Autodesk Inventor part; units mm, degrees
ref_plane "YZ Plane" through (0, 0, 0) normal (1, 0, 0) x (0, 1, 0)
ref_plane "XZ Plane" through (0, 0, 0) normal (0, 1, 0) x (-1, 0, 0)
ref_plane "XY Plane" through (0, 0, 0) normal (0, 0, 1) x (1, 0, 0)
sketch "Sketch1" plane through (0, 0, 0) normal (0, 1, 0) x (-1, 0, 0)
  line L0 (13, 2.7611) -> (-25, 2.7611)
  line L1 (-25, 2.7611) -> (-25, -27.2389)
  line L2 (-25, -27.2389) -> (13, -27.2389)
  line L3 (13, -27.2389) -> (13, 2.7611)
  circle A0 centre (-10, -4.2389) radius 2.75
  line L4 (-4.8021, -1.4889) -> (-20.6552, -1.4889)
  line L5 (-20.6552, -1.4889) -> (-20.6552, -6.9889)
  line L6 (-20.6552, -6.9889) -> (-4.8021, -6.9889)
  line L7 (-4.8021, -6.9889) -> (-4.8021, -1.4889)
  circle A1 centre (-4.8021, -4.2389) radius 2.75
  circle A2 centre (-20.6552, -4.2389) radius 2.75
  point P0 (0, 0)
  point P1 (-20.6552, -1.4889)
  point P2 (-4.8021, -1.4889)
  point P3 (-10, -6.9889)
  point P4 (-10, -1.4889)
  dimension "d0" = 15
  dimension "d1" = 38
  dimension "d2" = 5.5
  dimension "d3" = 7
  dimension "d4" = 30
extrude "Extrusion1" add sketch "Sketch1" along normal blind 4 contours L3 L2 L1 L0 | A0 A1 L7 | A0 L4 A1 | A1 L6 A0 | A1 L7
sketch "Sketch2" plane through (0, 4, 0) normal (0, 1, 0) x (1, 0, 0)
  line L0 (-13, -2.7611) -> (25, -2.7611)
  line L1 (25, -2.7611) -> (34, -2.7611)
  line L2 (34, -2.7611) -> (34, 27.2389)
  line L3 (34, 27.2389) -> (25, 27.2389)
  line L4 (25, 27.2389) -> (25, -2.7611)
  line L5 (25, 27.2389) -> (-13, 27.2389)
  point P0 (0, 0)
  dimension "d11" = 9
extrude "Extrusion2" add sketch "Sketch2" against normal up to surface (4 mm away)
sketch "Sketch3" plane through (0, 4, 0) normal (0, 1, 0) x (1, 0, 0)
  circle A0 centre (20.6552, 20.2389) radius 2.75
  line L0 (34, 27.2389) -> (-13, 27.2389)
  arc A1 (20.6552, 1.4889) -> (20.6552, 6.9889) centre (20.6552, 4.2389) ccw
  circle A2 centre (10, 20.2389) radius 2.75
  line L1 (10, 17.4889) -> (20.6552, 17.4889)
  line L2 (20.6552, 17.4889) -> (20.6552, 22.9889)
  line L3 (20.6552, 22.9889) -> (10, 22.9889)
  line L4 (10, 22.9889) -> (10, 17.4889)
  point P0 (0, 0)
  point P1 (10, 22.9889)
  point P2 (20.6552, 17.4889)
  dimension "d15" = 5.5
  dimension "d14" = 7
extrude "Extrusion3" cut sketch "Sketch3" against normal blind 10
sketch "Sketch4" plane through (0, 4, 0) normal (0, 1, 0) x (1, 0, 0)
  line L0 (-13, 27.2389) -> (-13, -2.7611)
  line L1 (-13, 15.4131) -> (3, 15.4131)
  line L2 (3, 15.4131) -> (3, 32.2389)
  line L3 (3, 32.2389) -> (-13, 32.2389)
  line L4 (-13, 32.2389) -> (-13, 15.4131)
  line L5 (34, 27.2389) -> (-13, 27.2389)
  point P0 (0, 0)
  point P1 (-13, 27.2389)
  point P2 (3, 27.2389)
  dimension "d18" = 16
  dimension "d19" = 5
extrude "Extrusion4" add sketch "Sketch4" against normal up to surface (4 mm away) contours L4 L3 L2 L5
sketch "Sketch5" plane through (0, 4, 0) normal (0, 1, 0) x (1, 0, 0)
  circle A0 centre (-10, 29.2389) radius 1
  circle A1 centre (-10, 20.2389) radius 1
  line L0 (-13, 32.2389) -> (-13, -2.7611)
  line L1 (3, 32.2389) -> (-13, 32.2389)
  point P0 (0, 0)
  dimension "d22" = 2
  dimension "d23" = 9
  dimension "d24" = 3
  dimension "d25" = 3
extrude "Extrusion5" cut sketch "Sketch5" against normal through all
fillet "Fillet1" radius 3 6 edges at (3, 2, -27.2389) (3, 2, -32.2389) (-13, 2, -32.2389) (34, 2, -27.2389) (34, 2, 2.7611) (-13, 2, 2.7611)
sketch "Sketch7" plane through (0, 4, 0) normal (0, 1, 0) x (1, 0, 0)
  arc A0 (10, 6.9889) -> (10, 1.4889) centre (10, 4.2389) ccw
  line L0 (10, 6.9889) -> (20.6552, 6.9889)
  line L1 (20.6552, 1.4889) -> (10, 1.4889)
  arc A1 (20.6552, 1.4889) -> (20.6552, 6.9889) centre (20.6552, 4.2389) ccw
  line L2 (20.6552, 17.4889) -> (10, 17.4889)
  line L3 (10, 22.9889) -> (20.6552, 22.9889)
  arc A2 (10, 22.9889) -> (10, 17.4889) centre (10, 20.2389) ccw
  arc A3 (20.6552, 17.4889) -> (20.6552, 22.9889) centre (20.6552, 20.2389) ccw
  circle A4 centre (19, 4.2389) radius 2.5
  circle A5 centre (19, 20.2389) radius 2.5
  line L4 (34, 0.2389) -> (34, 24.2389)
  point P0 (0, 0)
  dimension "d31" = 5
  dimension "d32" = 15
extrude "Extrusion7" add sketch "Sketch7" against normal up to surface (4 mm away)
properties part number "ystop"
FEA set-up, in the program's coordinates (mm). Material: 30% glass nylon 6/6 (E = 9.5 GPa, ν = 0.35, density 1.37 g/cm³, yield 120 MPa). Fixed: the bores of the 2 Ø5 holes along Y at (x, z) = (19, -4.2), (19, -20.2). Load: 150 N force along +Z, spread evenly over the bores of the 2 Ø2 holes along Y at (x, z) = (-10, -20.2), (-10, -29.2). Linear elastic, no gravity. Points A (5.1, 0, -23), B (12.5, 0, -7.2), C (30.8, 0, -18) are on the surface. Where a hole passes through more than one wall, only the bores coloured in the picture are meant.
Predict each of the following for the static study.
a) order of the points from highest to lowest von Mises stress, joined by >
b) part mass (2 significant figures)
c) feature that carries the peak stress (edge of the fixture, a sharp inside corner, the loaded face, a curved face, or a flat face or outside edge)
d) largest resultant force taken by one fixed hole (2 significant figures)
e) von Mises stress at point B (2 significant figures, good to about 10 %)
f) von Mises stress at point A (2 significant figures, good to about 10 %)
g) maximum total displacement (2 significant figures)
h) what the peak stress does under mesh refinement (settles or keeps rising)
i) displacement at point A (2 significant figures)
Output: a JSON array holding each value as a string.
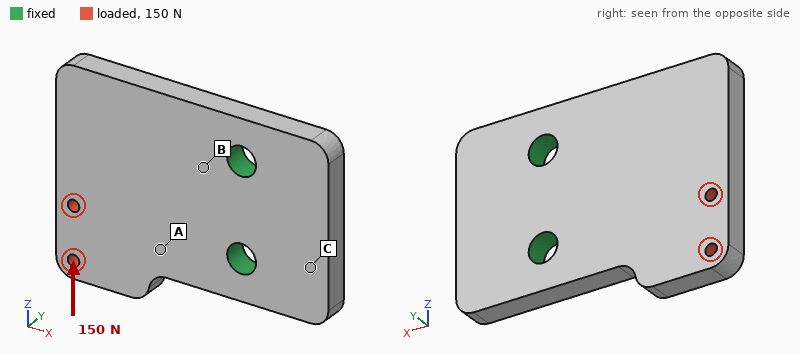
["B > A > C", "7.9 g", "edge of the fixture", "240 N", "4.6 MPa", "2.7 MPa", "40 µm", "keeps rising", "13 µm"]
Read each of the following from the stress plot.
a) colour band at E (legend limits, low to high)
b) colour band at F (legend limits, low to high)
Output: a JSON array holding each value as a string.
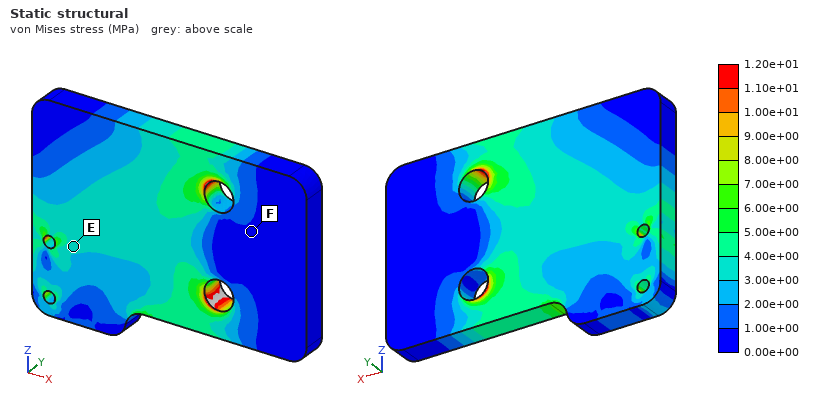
["3.00e+00 to 4.00e+00 MPa", "0.00e+00 to 1.00e+00 MPa"]
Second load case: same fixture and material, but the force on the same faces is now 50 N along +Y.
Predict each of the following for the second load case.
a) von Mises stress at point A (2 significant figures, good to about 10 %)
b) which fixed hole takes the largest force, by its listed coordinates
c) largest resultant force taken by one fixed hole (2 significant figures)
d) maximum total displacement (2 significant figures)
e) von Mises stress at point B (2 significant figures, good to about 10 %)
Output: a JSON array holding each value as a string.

["12 MPa", "(19, -20.2)", "55 N", "0.37 mm", "11 MPa"]
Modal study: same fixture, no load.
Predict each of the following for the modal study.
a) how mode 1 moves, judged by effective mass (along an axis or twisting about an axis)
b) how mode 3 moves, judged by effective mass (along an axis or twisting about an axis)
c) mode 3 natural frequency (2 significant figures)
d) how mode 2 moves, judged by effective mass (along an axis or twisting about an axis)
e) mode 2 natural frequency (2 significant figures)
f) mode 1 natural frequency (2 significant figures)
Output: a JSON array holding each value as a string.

["along Y", "along Z", "7300 Hz", "twisting about X", "3500 Hz", "1700 Hz"]
